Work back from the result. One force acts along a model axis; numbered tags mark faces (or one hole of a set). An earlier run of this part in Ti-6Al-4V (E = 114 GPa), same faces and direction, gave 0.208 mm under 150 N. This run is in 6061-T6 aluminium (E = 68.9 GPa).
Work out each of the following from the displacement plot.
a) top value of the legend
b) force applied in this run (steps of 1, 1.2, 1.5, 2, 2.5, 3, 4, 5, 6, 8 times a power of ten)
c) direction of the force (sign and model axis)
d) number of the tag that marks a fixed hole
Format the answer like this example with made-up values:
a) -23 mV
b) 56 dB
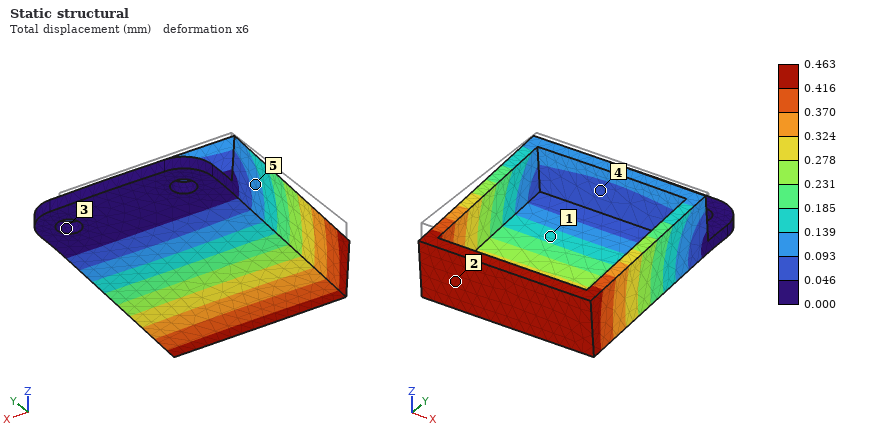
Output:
a) 0.463 mm
b) 200 N
c) -Z
d) 3
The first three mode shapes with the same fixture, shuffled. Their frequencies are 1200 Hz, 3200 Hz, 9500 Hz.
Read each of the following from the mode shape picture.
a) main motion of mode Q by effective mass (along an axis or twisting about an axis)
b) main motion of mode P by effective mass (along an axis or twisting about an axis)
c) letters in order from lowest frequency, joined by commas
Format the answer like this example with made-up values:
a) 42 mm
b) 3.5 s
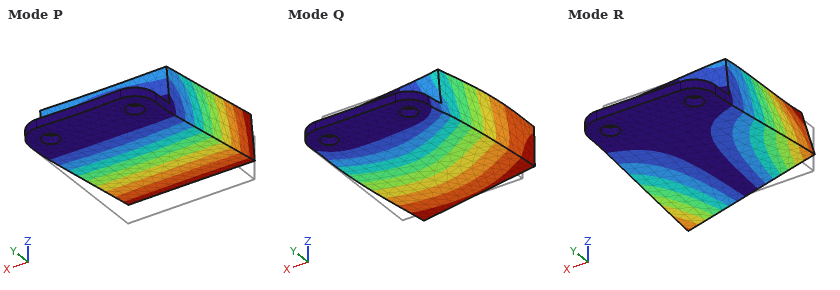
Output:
a) along X
b) along Z
c) P, R, Q
